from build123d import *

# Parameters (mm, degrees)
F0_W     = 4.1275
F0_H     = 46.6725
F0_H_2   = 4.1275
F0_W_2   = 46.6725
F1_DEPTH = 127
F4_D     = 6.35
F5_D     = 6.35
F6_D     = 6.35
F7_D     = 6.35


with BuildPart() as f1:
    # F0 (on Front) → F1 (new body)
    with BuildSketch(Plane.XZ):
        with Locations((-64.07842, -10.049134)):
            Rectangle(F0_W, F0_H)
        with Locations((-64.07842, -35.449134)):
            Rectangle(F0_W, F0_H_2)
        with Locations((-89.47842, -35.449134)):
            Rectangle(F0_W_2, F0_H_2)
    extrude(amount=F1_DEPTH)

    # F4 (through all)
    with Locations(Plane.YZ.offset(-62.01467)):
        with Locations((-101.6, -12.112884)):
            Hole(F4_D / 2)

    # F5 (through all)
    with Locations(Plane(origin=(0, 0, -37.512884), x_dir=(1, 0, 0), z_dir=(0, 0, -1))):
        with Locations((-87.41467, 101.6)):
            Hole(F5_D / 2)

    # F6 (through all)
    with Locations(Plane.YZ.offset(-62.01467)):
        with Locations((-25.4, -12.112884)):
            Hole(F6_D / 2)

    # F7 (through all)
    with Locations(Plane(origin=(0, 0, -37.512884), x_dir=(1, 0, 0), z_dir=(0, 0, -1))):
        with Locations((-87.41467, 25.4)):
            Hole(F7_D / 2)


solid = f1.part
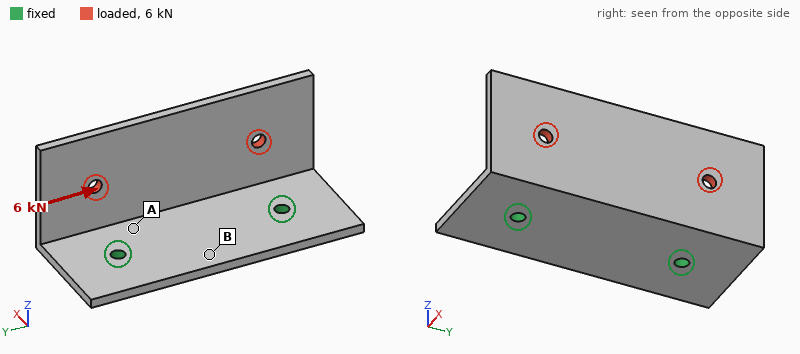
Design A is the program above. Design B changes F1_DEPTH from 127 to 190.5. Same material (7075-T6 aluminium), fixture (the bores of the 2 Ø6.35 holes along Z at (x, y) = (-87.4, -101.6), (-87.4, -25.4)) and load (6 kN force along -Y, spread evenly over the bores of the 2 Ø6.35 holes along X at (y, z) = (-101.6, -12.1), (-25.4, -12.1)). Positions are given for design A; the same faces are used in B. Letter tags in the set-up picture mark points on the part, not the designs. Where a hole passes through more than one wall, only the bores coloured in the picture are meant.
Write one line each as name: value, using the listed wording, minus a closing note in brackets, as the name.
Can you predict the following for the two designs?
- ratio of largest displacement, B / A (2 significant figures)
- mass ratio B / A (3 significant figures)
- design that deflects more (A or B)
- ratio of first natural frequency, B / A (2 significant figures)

ratio of largest displacement, B / A: 1.4
mass ratio B / A: 1.51
design that deflects more: B
ratio of first natural frequency, B / A: 0.79
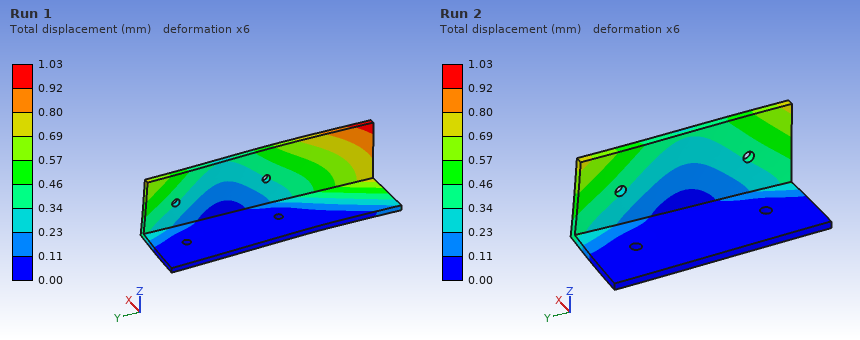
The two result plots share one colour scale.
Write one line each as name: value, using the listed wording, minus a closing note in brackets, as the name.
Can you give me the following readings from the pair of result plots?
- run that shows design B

run that shows design B: Run 1
